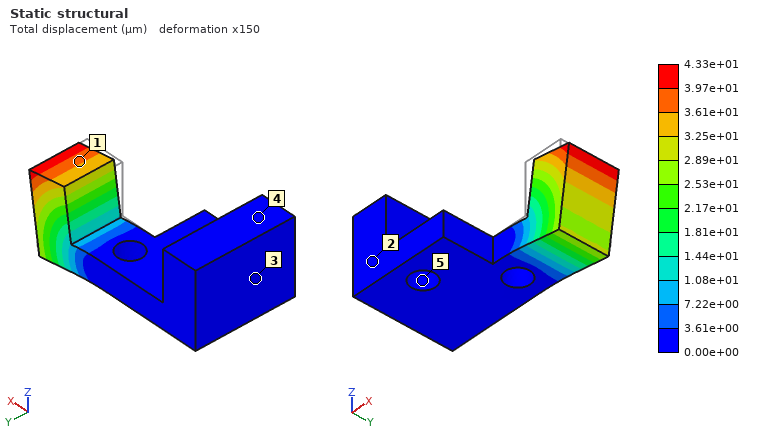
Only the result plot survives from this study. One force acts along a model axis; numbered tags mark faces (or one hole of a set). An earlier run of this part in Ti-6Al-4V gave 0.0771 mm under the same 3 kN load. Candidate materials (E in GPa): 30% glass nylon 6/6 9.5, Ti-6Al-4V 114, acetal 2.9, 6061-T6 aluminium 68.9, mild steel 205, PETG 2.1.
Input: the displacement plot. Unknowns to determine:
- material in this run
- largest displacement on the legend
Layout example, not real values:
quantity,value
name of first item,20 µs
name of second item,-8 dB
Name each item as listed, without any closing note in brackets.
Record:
quantity,value
material in this run,mild steel
largest displacement on the legend,4.33e+01 µm
